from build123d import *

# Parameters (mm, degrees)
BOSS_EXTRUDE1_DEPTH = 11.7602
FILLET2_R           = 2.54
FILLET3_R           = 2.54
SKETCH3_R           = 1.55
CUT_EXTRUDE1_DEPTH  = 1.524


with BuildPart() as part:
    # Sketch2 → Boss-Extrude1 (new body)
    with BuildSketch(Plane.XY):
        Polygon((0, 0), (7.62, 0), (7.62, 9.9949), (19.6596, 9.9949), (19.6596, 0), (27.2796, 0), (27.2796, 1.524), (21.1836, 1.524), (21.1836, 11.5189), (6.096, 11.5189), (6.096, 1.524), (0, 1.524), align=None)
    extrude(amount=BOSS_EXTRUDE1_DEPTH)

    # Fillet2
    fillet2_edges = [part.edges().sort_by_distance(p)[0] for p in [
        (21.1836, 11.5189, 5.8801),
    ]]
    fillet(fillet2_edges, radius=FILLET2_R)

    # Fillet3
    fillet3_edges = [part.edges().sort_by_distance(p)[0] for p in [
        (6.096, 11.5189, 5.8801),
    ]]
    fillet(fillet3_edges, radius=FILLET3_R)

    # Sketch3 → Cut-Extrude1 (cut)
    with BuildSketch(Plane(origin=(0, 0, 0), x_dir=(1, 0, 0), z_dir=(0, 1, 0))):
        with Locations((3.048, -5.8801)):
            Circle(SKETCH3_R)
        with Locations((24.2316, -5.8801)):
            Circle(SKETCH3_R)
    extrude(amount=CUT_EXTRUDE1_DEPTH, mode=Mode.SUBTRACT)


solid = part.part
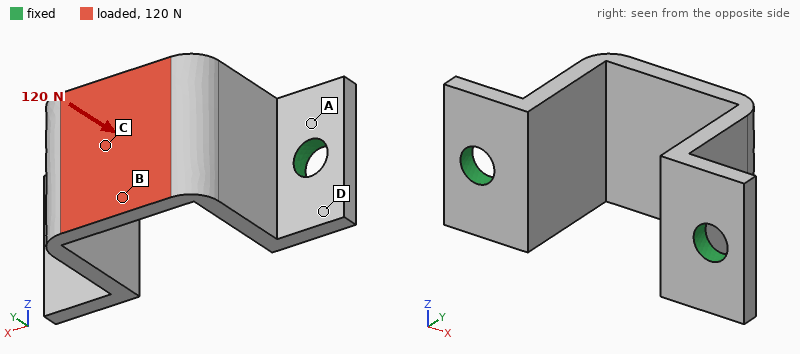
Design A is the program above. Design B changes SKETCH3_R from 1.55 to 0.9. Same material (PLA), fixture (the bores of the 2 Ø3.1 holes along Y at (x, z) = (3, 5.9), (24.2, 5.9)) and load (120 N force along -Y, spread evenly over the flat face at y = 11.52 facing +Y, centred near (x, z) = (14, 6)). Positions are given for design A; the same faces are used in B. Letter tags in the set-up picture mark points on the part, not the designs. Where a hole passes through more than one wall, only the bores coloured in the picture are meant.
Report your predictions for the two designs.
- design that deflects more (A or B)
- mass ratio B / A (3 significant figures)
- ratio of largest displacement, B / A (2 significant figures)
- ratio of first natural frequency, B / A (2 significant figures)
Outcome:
B
1.02
1.1
0.78
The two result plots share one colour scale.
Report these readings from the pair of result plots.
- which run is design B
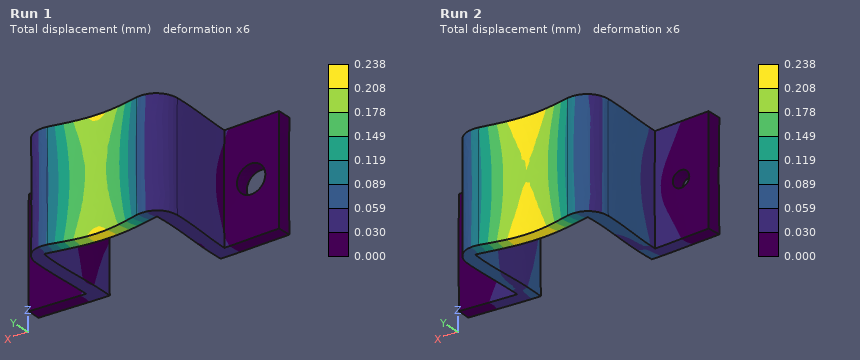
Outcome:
Run 2
